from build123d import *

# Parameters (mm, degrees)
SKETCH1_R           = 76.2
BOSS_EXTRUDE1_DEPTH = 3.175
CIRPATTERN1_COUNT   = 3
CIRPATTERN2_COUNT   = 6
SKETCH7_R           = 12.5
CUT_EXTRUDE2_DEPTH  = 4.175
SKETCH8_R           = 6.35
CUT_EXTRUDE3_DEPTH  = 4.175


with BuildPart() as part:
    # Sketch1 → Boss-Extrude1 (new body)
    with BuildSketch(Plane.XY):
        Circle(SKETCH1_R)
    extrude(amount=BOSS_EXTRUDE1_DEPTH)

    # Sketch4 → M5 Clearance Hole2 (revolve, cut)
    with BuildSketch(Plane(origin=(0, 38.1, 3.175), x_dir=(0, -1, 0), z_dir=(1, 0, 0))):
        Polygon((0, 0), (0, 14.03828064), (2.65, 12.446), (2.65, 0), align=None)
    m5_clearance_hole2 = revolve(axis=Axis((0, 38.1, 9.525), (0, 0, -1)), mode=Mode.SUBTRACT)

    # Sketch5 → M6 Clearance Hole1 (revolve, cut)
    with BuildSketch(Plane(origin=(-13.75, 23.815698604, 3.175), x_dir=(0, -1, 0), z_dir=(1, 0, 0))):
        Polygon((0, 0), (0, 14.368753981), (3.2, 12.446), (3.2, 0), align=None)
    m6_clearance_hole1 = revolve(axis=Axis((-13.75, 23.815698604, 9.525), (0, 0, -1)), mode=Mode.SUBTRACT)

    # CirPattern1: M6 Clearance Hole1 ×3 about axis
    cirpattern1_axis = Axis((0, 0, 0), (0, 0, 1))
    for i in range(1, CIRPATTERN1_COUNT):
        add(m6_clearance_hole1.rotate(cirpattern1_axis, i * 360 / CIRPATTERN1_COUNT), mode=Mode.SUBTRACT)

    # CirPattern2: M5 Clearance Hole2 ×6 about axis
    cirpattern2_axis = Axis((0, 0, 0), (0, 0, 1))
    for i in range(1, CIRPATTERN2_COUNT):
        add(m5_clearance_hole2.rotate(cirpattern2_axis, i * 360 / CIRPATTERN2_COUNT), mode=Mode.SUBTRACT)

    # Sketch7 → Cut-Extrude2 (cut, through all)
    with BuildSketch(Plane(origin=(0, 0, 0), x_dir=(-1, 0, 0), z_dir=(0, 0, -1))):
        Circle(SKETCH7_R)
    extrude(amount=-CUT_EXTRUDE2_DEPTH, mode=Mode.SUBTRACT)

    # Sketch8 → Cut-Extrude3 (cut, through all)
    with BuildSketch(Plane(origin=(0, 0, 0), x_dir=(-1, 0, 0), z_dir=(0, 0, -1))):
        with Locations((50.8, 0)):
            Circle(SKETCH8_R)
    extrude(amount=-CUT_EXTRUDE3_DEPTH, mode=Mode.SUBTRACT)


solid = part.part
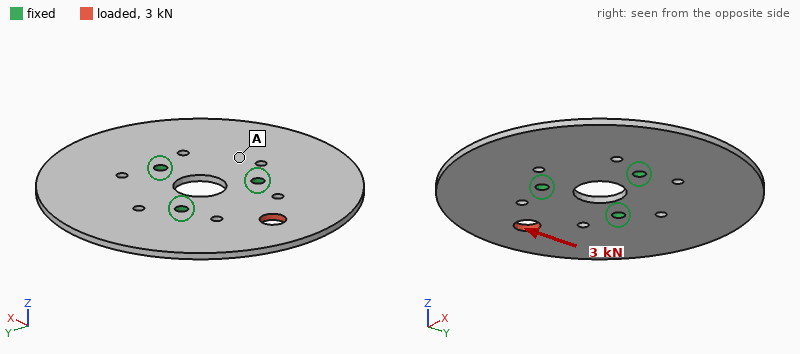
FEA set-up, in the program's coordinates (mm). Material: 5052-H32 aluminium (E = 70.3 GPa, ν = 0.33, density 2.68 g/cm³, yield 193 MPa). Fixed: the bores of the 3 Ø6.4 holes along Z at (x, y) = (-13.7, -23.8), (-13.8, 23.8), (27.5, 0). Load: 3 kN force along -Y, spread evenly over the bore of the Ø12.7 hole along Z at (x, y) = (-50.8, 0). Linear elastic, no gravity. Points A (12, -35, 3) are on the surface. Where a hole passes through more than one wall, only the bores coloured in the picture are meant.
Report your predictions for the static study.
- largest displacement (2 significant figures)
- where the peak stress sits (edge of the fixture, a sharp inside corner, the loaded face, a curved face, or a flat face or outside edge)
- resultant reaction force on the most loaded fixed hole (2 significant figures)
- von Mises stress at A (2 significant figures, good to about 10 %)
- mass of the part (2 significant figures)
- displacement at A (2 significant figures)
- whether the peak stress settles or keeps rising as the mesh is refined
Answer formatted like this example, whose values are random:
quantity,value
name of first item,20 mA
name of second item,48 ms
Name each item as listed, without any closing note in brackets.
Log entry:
quantity,value
largest displacement,30 µm
where the peak stress sits,edge of the fixture
resultant reaction force on the most loaded fixed hole,2.4 kN
von Mises stress at A,7.2 MPa
mass of the part,150 g
displacement at A,5.2 µm
whether the peak stress settles or keeps rising as the mesh is refined,keeps rising
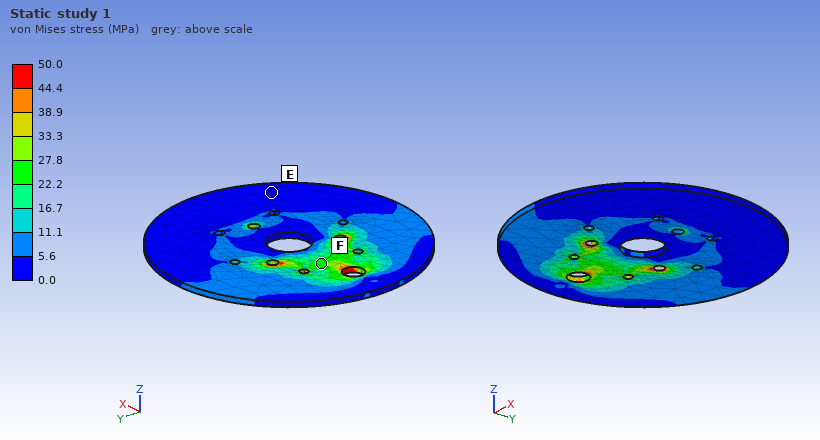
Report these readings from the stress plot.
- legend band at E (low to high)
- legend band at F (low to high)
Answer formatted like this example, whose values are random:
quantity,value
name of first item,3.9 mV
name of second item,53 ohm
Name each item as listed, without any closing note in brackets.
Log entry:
quantity,value
legend band at E,0.0 to 5.6 MPa
legend band at F,22.2 to 27.8 MPa
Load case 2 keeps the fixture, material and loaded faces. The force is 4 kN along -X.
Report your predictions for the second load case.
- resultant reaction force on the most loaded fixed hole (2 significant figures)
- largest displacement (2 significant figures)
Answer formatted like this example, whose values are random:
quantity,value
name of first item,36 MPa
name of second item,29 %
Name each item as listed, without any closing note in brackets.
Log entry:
quantity,value
resultant reaction force on the most loaded fixed hole,2.0 kN
largest displacement,22 µm
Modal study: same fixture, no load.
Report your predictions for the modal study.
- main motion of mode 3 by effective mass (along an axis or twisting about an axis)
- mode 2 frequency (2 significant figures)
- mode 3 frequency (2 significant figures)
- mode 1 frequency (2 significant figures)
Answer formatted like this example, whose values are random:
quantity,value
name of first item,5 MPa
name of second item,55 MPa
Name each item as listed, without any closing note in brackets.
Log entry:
quantity,value
main motion of mode 3 by effective mass,along Z
mode 2 frequency,780 Hz
mode 3 frequency,900 Hz
mode 1 frequency,780 Hz
